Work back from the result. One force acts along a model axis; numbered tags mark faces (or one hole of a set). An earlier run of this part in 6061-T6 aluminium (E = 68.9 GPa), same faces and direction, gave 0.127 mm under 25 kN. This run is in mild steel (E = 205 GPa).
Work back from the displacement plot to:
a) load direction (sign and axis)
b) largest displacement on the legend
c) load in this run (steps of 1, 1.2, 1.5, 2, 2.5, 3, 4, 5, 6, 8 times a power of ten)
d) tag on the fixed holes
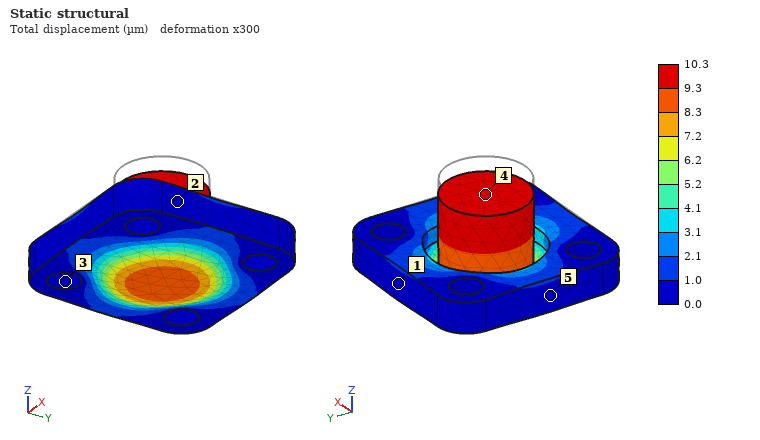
-Z
10.3 µm
6 kN
3
